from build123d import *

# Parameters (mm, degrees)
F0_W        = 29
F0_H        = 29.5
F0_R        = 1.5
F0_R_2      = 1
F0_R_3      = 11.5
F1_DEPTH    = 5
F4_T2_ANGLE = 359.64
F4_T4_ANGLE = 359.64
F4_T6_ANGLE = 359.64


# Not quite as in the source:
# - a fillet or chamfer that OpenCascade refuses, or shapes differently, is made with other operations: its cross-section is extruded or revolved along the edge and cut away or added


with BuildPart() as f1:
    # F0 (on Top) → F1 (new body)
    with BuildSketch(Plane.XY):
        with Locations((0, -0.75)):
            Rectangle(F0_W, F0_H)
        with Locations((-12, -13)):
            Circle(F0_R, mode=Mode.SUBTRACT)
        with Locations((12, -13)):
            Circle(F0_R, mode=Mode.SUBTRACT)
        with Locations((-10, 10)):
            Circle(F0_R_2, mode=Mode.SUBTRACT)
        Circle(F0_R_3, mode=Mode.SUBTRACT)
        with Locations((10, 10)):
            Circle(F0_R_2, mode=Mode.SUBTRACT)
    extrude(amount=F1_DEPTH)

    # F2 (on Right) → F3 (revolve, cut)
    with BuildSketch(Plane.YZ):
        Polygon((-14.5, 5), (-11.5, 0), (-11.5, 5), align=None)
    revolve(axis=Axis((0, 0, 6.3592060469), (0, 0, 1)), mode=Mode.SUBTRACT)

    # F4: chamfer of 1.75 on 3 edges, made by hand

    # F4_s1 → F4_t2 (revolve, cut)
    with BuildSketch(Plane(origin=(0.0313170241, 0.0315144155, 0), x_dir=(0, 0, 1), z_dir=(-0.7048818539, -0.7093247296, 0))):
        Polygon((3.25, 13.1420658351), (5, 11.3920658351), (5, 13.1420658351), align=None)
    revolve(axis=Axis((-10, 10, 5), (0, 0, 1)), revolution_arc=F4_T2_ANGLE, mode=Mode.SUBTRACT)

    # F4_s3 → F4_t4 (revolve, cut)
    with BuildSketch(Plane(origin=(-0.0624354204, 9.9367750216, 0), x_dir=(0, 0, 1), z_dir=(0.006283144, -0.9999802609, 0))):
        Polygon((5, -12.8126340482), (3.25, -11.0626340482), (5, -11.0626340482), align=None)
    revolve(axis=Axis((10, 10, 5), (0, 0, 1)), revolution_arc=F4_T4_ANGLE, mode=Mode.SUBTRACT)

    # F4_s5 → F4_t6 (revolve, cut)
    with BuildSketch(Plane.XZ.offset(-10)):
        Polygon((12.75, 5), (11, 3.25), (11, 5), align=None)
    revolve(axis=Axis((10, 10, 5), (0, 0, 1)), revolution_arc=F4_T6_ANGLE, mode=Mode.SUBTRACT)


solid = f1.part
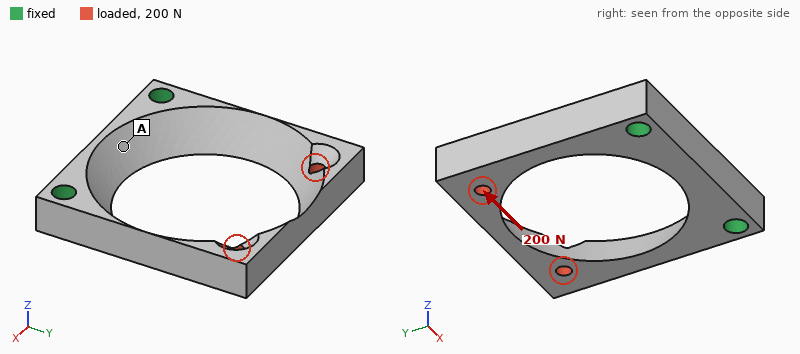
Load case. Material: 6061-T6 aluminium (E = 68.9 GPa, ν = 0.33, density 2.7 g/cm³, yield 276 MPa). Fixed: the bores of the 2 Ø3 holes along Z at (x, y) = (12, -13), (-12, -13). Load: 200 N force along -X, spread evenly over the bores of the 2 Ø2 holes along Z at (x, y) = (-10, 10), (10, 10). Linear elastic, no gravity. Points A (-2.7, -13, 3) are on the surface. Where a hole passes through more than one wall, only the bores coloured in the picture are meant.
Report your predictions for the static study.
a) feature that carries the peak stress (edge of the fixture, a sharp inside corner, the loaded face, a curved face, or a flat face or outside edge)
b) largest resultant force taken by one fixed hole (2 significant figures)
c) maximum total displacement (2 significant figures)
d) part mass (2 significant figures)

the loaded face
140 N
0.13 mm
4.0 g
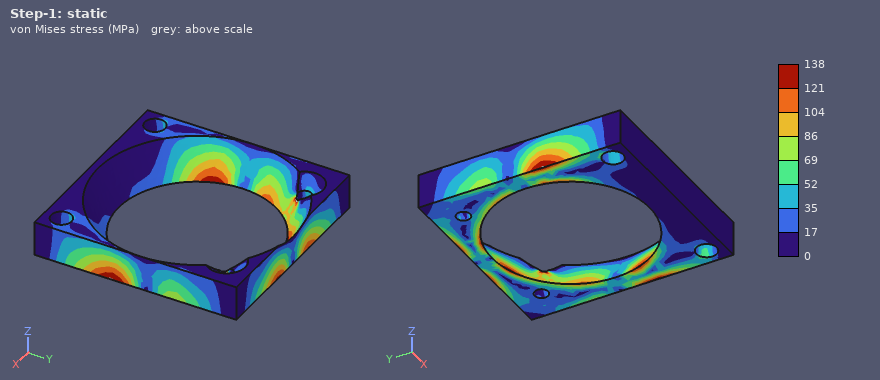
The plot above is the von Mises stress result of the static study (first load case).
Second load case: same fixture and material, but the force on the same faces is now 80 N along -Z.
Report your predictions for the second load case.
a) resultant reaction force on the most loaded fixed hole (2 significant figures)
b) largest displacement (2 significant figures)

42 N
0.14 mm
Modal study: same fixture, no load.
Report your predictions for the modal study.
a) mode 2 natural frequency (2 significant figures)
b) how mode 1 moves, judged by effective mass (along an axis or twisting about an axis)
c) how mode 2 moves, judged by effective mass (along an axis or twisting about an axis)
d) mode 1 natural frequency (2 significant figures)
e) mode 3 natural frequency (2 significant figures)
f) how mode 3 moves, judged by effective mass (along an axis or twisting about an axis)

4600 Hz
along Z
along X
3400 Hz
6500 Hz
along X
